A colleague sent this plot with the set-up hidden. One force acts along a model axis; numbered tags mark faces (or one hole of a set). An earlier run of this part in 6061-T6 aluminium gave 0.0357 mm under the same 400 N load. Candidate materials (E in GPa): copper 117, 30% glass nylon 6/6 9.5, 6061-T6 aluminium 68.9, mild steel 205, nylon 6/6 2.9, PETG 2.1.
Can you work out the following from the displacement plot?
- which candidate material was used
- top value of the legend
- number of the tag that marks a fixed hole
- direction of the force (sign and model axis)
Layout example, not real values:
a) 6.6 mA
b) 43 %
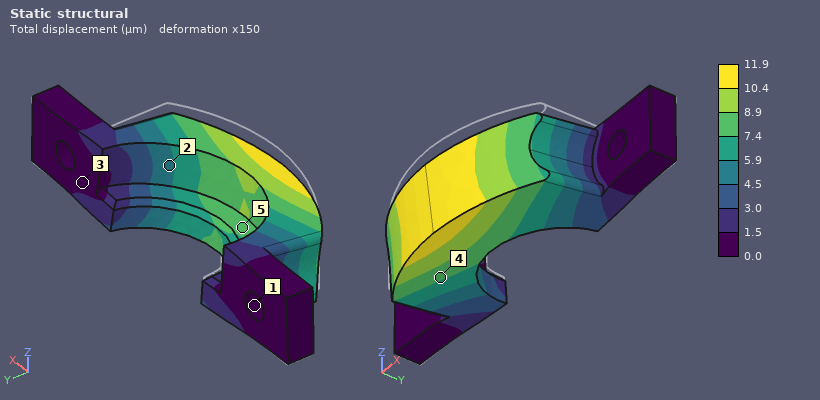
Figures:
a) mild steel
b) 11.9 µm
c) 1
d) -Z
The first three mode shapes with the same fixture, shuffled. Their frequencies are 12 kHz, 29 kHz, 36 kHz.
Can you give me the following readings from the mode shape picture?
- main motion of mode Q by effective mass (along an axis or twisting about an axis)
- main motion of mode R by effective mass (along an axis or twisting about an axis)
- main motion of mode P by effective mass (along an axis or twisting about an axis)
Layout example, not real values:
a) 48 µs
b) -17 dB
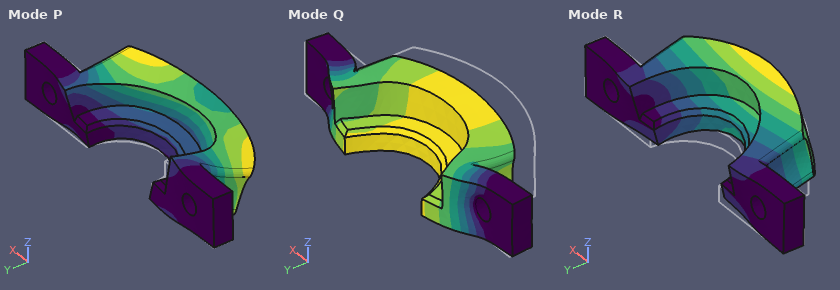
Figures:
a) along Y
b) along Z
c) along X
